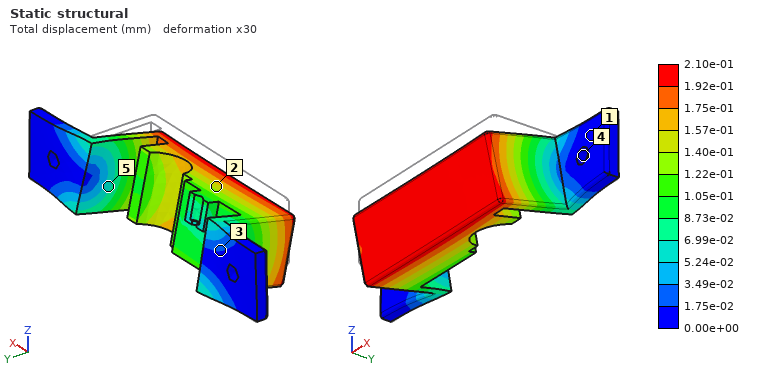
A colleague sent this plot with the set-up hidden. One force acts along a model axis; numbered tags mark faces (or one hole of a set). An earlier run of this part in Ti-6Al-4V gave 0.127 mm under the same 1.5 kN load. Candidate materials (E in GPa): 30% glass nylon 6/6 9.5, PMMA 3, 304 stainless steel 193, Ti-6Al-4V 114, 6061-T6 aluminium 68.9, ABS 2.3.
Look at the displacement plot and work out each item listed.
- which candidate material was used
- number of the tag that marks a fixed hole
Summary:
6061-T6 aluminium
4
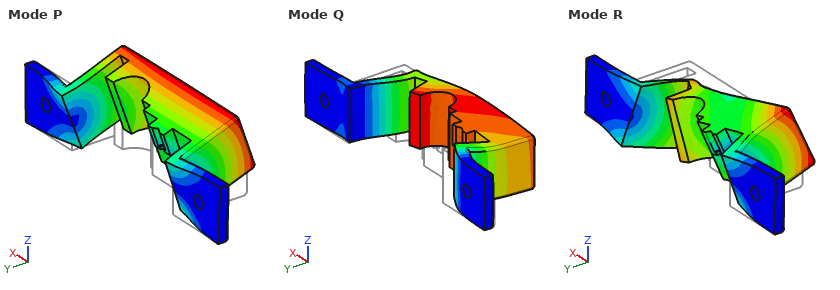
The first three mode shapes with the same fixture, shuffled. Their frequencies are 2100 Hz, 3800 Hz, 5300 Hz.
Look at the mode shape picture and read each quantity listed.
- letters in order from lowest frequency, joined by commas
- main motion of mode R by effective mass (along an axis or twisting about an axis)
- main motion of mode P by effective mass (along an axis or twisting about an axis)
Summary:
P, Q, R
twisting about Y
along Z
